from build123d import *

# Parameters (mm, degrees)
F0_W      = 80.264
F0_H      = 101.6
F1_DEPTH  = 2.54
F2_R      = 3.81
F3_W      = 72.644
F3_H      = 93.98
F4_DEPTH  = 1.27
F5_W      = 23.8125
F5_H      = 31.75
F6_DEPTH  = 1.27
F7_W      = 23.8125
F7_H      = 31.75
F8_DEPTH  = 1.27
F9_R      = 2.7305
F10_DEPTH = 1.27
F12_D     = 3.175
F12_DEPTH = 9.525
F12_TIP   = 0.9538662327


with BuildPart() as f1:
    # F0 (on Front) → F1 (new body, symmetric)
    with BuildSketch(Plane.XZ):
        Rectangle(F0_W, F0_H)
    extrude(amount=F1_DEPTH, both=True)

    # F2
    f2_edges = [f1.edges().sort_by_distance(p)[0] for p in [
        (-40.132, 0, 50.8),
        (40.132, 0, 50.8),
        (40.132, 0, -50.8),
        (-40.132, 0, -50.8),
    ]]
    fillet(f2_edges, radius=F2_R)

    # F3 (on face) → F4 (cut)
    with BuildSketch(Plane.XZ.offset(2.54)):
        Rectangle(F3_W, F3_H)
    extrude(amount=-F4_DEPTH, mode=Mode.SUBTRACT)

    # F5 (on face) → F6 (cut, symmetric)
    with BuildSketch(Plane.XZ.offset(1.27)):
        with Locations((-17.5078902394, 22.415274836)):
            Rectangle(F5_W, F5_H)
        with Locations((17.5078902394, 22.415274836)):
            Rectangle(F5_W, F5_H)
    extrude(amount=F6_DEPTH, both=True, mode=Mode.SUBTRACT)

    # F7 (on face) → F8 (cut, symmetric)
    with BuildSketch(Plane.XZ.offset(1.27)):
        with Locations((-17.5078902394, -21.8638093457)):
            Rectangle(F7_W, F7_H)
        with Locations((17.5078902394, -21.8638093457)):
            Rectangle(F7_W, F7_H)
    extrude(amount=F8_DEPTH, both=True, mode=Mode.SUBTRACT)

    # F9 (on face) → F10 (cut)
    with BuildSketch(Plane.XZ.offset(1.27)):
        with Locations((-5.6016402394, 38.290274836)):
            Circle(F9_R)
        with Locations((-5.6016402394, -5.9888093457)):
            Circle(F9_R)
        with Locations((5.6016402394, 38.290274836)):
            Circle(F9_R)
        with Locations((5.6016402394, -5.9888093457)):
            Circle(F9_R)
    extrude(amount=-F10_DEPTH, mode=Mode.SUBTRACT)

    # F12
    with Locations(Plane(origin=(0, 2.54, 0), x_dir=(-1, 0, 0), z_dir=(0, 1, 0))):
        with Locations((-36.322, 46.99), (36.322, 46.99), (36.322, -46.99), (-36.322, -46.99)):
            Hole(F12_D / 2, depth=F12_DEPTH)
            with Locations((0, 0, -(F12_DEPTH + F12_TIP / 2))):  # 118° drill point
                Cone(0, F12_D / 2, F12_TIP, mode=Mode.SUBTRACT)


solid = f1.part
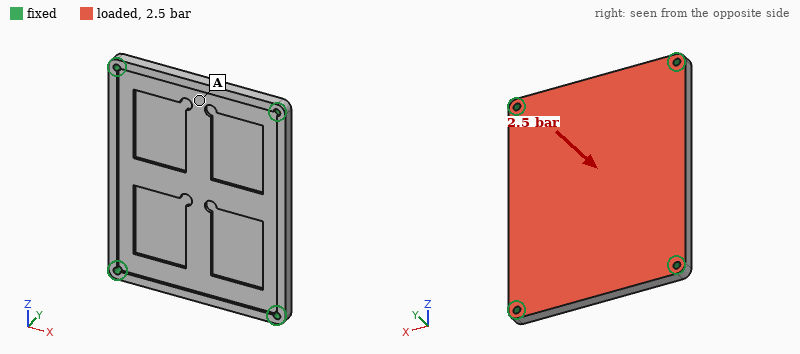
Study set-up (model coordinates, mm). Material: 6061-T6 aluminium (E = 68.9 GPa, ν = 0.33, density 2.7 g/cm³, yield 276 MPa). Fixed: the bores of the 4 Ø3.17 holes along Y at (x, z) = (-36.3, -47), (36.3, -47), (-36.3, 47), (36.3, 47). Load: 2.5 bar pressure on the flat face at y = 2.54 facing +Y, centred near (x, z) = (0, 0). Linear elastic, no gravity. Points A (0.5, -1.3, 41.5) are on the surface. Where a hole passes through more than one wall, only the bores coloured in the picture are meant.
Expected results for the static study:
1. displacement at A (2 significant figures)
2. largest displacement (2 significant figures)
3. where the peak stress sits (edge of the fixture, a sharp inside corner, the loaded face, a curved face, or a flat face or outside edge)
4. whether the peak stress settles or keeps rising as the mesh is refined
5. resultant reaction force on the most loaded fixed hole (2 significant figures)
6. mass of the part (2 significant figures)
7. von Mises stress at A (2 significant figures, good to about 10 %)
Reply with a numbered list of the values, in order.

1. 0.13 mm
2. 0.35 mm
3. edge of the fixture
4. keeps rising
5. 720 N
6. 77 g
7. 30 MPa
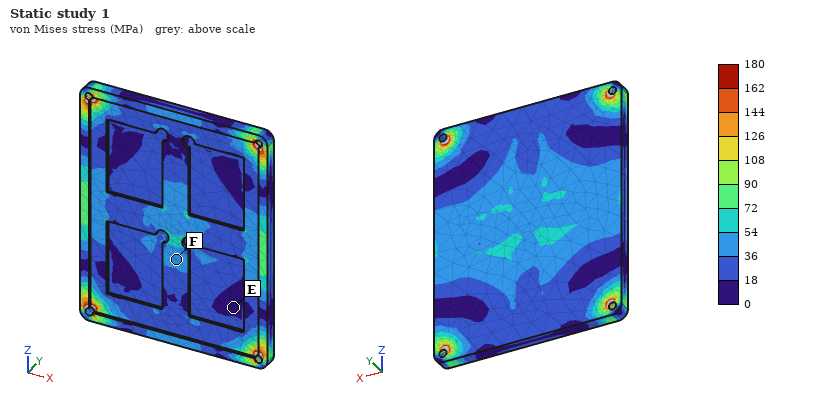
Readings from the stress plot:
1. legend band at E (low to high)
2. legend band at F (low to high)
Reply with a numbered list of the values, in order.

1. 0 to 18 MPa
2. 36 to 54 MPa
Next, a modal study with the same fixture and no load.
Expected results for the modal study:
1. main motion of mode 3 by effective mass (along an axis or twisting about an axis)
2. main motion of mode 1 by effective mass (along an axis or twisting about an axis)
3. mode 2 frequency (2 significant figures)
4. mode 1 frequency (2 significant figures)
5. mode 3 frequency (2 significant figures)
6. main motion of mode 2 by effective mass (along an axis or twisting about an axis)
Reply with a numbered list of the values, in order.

1. twisting about X
2. along Y
3. 2700 Hz
4. 1700 Hz
5. 3600 Hz
6. twisting about Z
